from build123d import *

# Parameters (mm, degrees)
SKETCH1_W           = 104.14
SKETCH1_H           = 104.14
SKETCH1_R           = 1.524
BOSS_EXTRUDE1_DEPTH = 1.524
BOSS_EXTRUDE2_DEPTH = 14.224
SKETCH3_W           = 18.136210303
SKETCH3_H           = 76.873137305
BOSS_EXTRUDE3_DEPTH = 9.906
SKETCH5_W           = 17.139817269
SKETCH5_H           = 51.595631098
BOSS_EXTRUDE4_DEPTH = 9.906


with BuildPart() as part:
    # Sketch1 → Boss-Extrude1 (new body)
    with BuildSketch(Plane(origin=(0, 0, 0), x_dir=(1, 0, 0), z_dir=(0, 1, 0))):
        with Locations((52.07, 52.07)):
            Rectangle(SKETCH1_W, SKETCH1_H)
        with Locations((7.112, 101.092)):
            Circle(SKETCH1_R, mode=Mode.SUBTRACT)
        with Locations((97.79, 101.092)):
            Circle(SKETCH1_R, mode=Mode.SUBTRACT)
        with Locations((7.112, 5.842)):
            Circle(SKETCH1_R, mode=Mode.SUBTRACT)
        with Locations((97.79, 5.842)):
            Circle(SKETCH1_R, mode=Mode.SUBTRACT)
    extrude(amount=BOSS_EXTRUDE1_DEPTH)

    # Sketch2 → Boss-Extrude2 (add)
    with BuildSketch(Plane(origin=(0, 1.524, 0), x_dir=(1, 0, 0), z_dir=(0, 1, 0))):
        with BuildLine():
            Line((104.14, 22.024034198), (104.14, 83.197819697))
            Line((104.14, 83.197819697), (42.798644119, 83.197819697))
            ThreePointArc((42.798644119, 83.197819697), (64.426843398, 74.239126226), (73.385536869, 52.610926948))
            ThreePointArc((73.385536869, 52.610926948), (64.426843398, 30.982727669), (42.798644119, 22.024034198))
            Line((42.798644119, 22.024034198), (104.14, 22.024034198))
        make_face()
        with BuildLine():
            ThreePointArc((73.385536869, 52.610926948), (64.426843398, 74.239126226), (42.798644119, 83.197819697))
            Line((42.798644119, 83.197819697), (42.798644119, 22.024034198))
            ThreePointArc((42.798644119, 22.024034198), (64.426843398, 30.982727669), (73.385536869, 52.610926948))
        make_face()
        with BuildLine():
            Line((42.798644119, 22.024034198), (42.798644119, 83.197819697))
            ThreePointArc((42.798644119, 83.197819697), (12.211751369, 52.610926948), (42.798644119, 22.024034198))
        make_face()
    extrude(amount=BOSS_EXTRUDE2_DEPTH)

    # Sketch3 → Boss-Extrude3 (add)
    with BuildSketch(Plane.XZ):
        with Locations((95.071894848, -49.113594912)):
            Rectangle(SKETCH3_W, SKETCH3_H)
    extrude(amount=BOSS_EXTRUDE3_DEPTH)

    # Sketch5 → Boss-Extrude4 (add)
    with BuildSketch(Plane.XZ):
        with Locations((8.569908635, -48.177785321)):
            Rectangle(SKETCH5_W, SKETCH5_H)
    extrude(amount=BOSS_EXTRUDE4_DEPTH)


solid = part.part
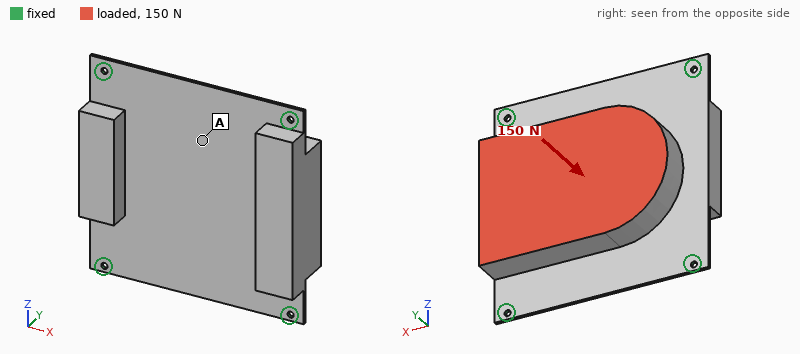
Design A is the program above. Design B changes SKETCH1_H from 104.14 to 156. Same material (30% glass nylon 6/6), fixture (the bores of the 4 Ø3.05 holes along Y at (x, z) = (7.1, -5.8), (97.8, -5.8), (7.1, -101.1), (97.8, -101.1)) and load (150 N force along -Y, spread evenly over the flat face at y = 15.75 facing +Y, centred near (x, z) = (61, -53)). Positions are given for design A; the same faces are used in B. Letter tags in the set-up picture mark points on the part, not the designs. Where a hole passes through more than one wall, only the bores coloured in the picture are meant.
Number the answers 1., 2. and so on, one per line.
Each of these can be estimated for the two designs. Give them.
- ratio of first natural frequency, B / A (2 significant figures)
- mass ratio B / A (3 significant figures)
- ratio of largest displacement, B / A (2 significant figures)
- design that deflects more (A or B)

1. 1.0
2. 1.07
3. 0.90
4. A
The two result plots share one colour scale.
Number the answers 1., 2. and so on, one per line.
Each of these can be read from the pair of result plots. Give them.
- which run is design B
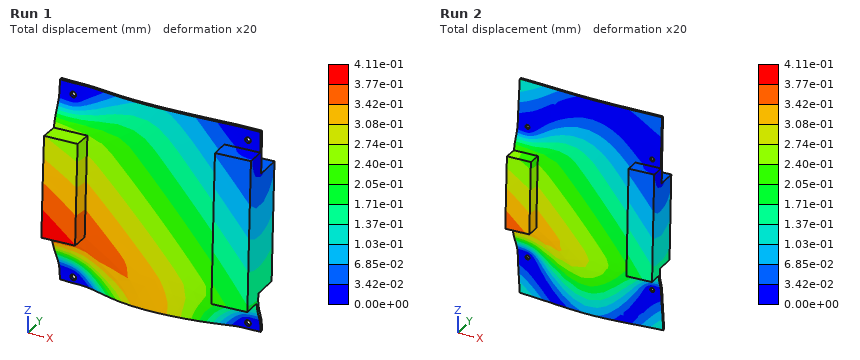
1. Run 2
